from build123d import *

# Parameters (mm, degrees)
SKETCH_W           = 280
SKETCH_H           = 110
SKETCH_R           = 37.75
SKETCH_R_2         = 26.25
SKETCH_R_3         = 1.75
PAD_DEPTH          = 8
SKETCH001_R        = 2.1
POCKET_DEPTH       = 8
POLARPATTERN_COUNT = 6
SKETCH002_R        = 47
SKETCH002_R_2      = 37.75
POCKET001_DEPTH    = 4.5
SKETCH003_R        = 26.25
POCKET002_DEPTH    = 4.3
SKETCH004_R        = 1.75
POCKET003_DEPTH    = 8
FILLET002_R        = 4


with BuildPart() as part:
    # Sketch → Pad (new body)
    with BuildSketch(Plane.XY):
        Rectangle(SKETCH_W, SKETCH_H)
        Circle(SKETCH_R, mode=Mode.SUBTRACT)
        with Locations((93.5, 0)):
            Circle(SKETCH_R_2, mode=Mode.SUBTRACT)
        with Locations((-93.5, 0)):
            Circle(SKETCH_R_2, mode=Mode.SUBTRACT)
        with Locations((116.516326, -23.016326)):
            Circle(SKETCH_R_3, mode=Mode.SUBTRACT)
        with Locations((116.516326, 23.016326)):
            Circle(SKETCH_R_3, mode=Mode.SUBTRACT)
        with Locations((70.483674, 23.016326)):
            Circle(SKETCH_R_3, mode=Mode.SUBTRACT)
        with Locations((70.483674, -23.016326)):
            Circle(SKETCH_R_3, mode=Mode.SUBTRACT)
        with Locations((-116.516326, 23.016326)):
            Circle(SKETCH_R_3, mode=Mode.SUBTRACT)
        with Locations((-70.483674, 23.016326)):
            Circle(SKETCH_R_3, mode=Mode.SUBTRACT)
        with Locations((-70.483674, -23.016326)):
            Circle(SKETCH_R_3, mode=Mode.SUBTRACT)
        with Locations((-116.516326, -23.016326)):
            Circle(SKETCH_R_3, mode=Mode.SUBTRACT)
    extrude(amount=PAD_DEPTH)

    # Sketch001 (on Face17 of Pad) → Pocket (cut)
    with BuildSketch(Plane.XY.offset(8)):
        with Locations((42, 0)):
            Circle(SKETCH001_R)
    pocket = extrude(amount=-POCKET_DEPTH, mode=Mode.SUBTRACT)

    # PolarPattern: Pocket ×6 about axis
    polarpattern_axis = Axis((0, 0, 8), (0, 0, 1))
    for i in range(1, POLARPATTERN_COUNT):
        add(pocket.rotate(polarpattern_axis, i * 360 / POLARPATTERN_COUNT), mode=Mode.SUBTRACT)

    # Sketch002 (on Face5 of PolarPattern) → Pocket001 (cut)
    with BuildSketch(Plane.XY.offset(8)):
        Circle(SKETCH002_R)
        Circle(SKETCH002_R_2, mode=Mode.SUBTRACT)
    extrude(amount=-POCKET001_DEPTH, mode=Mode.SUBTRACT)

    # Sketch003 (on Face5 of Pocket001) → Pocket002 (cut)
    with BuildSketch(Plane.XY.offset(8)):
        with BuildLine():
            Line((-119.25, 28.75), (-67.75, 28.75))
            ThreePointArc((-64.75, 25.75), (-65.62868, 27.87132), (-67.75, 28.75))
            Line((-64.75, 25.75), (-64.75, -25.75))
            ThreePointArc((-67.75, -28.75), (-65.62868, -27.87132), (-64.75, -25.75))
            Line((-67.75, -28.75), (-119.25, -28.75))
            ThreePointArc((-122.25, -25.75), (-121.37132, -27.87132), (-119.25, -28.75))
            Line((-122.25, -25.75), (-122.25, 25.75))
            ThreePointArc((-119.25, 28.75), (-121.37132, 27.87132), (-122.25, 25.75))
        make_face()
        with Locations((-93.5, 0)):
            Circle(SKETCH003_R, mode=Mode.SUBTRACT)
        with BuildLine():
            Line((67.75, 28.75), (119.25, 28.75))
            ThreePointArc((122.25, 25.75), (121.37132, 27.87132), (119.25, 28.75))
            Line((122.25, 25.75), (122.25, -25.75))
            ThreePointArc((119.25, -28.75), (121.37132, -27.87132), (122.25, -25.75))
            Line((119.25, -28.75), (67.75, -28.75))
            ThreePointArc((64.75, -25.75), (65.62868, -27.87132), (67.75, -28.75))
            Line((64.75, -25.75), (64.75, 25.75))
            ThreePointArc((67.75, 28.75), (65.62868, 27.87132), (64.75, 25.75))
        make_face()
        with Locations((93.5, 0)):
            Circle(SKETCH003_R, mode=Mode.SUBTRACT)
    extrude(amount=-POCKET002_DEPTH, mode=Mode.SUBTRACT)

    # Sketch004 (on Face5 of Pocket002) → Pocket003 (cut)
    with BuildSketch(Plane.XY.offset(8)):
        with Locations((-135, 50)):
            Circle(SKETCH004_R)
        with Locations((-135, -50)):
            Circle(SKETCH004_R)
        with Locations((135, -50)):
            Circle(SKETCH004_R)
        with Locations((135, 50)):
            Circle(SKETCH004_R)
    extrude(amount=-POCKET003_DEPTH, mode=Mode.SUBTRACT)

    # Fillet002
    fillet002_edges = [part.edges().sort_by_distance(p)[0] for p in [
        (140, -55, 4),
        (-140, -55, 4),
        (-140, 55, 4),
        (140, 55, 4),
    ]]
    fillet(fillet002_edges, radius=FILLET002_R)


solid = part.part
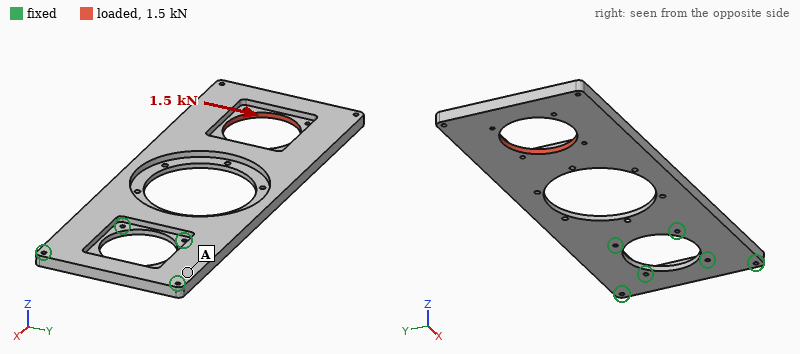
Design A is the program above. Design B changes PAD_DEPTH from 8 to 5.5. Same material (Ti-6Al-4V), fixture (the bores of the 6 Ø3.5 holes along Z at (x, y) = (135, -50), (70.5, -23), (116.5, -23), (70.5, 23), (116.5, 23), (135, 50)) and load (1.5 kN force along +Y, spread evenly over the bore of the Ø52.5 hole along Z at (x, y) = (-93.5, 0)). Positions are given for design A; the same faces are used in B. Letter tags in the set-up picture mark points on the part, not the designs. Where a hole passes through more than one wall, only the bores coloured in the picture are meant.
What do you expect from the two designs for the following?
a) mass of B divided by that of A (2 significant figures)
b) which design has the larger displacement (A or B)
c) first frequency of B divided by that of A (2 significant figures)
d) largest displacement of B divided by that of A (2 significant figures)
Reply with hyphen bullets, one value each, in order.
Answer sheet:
- 0.72
- B
- 0.71
- 1.3
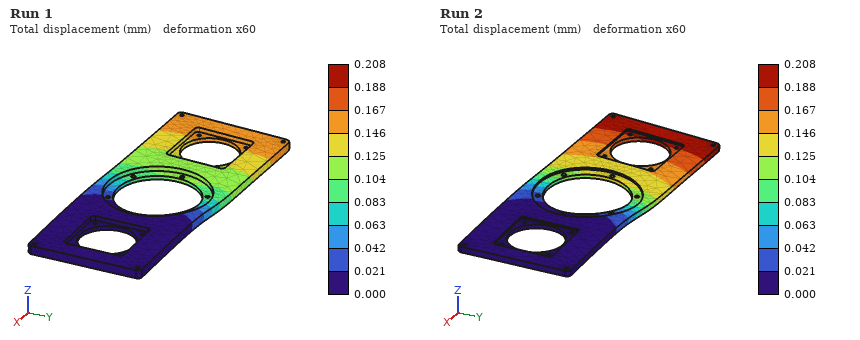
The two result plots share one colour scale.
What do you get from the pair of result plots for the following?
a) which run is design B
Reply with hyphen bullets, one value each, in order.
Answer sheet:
- Run 2
